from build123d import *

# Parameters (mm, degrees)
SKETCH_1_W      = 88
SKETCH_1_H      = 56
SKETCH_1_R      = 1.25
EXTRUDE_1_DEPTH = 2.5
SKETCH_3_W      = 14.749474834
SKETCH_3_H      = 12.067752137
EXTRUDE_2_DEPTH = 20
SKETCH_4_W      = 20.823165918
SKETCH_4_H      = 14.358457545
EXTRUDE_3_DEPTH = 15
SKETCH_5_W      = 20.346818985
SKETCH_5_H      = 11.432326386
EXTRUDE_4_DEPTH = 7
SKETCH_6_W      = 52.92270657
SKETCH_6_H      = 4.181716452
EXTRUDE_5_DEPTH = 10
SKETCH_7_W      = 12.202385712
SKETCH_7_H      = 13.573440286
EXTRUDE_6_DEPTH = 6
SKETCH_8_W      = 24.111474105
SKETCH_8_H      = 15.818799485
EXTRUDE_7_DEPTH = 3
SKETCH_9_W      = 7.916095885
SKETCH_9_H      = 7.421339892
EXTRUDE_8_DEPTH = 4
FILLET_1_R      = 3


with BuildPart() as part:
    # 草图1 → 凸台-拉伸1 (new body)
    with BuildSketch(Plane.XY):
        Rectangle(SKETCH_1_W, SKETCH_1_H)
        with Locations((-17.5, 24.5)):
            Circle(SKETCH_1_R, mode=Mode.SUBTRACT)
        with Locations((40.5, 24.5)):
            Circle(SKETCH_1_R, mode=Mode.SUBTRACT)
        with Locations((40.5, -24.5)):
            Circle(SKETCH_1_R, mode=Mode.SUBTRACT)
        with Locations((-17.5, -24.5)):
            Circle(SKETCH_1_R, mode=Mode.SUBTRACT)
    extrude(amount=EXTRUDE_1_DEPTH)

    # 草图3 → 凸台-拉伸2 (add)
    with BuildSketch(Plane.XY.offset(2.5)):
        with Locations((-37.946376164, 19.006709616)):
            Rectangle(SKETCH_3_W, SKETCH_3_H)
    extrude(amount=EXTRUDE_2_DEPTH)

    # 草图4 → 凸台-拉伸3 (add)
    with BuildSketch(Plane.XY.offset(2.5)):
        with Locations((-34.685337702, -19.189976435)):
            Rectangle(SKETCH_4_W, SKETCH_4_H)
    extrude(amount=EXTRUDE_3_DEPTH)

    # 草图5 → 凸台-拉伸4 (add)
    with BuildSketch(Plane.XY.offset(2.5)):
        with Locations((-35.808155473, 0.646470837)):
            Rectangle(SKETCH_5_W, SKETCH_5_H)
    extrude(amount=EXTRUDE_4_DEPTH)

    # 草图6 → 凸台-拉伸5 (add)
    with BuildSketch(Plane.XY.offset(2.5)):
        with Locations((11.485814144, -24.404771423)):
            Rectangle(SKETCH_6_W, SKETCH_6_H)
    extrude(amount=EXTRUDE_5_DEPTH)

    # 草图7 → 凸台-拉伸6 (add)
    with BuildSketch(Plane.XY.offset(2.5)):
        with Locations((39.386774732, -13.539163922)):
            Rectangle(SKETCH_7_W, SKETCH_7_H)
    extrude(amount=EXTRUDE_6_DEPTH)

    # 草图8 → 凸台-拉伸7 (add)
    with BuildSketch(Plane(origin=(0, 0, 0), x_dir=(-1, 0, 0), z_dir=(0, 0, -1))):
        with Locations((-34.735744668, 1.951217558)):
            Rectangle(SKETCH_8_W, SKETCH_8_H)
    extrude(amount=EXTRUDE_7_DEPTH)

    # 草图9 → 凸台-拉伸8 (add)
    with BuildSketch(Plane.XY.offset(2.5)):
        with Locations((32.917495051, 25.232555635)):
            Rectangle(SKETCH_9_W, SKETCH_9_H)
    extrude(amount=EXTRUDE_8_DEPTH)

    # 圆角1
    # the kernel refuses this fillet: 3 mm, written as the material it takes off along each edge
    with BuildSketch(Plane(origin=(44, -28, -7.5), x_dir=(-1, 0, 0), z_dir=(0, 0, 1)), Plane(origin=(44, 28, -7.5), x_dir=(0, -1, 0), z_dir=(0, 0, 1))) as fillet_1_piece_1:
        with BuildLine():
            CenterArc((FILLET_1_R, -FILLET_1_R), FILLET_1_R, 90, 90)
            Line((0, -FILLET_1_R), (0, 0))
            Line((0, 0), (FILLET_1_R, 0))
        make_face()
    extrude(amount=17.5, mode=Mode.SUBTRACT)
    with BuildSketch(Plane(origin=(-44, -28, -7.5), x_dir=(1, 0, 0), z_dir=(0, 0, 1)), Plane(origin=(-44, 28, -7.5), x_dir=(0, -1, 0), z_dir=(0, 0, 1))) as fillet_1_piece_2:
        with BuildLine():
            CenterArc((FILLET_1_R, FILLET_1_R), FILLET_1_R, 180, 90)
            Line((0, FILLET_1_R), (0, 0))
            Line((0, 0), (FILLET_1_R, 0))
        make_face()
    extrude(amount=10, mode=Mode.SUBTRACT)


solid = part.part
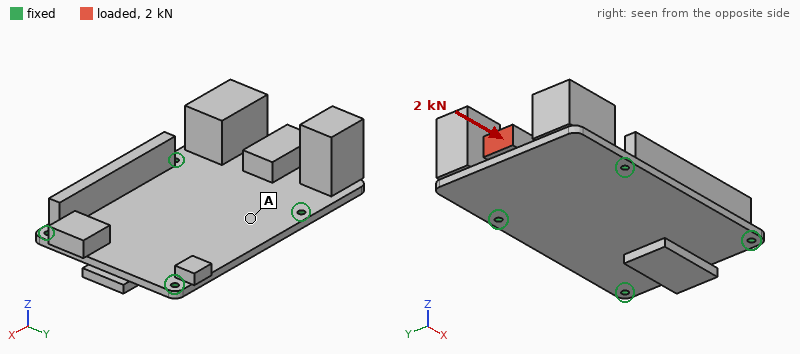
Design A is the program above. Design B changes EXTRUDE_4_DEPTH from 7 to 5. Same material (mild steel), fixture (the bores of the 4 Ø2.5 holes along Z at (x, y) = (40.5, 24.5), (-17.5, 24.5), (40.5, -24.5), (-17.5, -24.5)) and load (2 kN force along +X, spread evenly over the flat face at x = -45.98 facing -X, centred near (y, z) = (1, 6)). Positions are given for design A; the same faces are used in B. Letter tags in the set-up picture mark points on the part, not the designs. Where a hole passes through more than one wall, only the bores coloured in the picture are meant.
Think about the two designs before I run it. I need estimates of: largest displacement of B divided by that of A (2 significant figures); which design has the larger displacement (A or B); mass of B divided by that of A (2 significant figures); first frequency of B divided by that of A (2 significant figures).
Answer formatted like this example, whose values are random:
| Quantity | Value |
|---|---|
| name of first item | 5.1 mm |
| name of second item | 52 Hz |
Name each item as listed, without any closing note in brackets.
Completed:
| Quantity | Value |
|---|---|
| largest displacement of B divided by that of A | 0.80 |
| which design has the larger displacement | A |
| mass of B divided by that of A | 0.98 |
| first frequency of B divided by that of A | 1.0 |
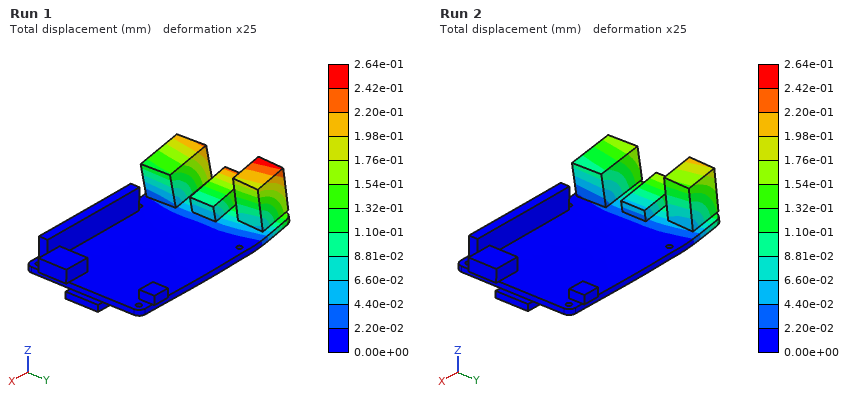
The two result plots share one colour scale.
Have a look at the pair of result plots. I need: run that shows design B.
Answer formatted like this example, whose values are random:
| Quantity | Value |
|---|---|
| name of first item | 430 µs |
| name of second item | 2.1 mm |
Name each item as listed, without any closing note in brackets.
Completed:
| Quantity | Value |
|---|---|
| run that shows design B | Run 2 |
